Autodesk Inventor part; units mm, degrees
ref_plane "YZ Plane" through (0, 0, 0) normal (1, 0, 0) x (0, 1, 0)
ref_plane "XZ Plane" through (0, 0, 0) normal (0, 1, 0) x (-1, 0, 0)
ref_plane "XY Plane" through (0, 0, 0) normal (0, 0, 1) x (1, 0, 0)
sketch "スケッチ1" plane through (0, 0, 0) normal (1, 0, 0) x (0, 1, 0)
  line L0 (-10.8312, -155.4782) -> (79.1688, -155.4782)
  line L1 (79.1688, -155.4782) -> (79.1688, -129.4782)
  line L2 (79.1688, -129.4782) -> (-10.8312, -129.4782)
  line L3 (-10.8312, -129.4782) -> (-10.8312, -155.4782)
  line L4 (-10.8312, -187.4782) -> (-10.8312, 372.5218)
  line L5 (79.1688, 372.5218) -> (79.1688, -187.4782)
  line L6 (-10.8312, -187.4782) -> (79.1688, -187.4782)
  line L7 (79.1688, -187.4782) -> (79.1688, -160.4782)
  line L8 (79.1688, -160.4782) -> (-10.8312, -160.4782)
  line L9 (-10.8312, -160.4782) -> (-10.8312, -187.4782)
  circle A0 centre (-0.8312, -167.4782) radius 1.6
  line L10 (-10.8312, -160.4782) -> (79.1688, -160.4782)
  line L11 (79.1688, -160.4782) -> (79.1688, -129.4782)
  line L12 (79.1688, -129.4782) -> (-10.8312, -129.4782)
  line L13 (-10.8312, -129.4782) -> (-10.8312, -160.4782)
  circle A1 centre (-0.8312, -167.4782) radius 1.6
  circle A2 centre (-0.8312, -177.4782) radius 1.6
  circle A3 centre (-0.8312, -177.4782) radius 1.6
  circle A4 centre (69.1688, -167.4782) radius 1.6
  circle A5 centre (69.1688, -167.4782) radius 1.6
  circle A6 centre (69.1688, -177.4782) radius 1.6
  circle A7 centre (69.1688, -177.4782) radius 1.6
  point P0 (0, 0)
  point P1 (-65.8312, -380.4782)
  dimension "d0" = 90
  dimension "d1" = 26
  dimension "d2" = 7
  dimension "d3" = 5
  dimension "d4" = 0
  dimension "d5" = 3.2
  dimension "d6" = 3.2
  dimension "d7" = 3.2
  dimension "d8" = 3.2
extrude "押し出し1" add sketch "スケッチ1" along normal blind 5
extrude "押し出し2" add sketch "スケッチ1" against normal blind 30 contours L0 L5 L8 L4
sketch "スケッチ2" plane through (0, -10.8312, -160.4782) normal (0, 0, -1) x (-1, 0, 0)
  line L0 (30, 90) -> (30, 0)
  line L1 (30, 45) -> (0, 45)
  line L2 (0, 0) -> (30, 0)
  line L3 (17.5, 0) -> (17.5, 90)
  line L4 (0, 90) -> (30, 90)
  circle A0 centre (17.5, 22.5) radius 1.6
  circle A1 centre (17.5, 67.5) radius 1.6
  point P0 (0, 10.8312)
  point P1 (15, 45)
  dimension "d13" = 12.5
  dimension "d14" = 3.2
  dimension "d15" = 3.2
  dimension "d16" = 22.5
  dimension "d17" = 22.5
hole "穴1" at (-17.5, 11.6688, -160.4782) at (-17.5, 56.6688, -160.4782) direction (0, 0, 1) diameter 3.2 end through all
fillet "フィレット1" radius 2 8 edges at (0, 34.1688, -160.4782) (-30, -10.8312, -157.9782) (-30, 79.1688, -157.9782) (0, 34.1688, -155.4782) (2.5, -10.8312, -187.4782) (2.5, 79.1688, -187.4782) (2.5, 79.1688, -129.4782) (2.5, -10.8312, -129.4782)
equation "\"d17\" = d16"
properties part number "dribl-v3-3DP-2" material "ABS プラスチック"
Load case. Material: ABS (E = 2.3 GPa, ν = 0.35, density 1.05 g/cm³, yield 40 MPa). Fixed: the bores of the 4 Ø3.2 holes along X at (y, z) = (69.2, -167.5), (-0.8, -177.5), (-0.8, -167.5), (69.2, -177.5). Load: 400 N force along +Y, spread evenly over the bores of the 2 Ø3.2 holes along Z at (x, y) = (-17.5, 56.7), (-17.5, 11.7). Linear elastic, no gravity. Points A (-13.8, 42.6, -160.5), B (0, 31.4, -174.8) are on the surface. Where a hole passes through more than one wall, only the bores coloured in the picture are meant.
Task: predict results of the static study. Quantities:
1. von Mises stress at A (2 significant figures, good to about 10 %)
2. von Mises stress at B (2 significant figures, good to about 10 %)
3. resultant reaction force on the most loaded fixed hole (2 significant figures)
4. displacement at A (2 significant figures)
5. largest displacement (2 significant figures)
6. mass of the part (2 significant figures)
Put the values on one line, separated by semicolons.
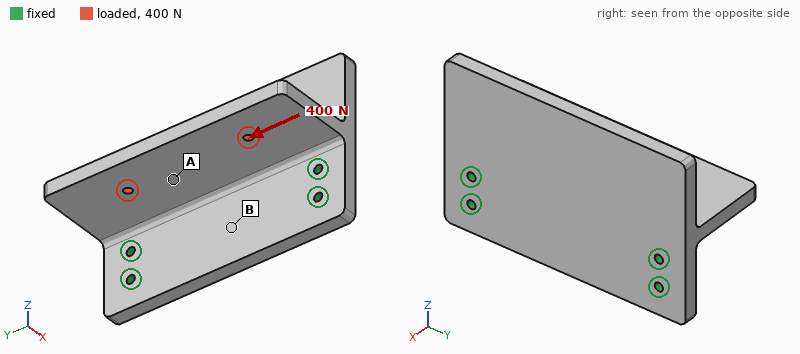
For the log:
2.4 MPa; 0.95 MPa; 200 N; 0.067 mm; 0.20 mm; 41 g
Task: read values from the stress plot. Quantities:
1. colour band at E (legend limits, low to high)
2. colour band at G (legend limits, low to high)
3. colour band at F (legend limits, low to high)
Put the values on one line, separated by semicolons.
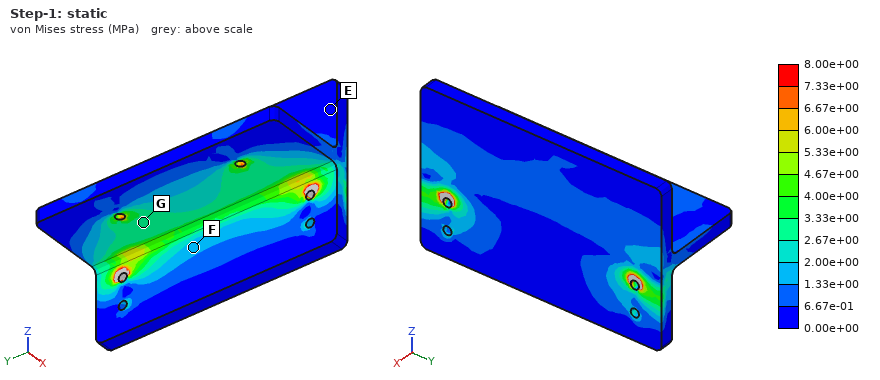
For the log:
0.00e+00 to 6.67e-01 MPa; 2.67e+00 to 3.33e+00 MPa; 1.33e+00 to 2.00e+00 MPa
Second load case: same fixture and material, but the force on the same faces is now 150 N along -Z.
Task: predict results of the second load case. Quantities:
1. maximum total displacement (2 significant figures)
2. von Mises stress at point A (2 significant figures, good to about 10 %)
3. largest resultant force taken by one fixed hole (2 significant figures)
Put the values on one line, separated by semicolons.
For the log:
0.83 mm; 1.7 MPa; 88 N
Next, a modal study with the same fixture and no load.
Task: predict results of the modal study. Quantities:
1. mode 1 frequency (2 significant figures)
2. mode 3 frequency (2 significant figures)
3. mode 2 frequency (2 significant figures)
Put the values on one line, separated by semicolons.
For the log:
550 Hz; 1400 Hz; 990 Hz
